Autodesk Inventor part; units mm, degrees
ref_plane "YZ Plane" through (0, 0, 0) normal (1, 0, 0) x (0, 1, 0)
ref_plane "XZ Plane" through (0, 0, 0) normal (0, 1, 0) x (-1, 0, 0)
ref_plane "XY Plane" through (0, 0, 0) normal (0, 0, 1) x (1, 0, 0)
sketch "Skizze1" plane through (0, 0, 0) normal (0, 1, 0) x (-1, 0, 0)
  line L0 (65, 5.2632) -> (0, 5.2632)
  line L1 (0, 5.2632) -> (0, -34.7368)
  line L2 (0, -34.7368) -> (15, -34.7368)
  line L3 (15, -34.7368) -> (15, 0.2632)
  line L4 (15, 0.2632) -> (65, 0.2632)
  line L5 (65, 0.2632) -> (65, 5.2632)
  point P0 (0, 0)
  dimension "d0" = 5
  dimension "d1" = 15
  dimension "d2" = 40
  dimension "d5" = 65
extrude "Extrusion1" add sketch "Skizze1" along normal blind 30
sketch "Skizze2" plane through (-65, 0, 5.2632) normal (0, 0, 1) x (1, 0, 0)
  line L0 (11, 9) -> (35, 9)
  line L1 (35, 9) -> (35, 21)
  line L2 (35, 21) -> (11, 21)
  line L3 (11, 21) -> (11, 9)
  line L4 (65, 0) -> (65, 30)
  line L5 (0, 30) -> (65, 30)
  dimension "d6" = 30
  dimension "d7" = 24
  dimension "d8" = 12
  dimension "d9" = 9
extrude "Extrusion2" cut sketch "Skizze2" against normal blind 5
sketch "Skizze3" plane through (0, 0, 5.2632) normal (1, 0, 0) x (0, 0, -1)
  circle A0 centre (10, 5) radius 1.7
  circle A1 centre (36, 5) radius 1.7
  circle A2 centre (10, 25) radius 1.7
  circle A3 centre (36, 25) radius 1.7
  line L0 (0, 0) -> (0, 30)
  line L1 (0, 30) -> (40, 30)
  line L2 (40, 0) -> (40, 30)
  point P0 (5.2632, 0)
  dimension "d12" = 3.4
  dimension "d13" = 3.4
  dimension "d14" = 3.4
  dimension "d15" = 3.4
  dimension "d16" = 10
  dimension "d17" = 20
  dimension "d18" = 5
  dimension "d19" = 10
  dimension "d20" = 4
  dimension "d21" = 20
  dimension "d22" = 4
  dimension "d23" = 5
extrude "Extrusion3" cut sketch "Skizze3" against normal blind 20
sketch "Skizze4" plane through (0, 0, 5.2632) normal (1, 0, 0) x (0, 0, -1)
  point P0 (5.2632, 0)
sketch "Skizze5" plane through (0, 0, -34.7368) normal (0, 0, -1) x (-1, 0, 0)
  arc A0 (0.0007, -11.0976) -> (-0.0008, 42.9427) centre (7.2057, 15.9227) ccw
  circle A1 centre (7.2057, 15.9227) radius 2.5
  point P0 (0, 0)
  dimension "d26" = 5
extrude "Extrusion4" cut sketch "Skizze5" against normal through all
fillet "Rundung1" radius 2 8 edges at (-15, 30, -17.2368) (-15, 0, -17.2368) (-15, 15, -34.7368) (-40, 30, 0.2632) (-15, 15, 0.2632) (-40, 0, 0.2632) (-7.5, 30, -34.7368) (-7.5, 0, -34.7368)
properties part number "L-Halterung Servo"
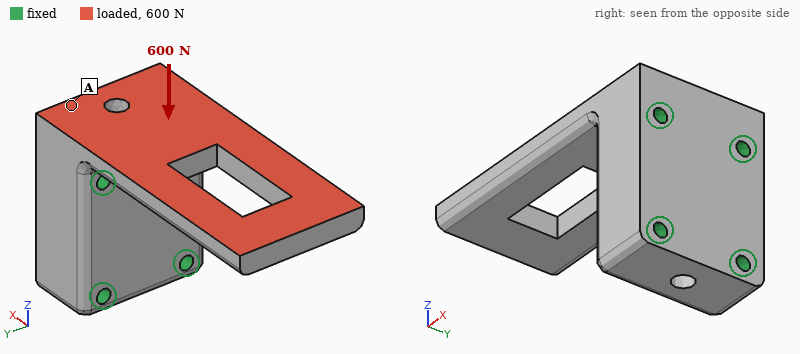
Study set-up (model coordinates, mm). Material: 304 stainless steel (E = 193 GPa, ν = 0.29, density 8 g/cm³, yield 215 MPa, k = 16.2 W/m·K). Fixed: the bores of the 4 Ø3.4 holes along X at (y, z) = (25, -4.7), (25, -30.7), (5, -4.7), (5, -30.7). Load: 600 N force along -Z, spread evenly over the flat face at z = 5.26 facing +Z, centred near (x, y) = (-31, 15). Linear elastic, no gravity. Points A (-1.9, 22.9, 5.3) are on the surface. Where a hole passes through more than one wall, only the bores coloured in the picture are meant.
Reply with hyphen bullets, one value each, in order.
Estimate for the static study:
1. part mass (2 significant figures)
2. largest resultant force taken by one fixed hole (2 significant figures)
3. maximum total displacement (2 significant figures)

- 180 g
- 290 N
- 0.17 mm
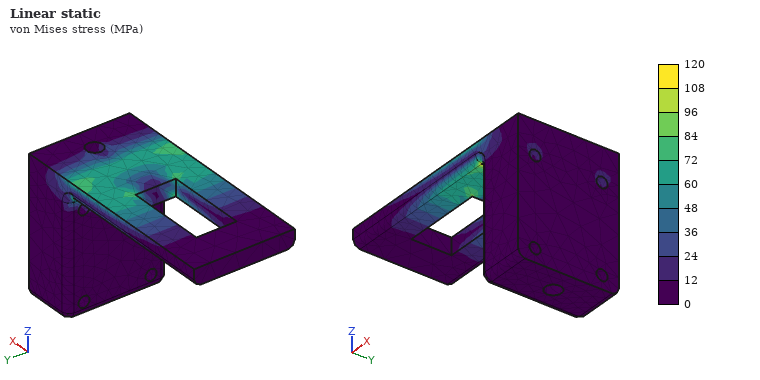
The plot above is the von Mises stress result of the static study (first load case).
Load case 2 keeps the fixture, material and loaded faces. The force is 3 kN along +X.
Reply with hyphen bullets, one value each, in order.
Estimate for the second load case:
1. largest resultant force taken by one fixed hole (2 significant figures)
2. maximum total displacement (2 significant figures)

- 1.6 kN
- 0.12 mm
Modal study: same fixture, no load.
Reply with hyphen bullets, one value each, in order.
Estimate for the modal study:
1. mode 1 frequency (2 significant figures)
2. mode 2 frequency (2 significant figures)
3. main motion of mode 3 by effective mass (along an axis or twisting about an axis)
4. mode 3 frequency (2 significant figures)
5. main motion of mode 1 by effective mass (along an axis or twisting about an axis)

- 1400 Hz
- 4400 Hz
- along Y
- 4800 Hz
- along Z
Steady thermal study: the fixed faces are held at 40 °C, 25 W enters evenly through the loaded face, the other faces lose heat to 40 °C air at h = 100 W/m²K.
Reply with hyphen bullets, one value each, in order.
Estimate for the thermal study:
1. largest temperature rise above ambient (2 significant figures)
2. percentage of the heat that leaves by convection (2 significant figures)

- 73 K
- 51 %
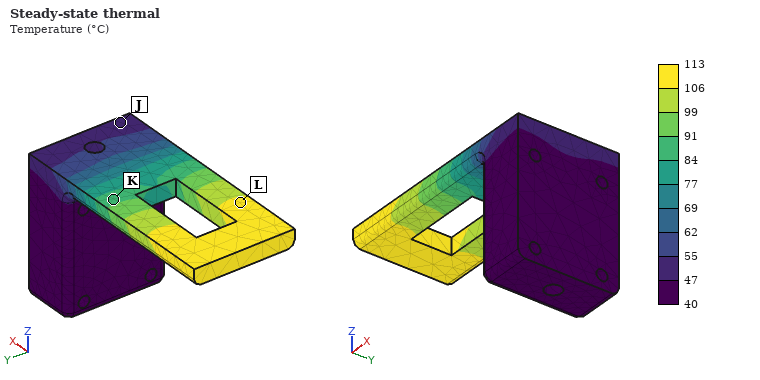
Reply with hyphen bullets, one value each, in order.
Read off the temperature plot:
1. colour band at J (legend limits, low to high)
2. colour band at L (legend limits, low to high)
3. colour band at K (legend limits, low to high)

- 47 to 55 °C
- 106 to 113 °C
- 84 to 91 °C
